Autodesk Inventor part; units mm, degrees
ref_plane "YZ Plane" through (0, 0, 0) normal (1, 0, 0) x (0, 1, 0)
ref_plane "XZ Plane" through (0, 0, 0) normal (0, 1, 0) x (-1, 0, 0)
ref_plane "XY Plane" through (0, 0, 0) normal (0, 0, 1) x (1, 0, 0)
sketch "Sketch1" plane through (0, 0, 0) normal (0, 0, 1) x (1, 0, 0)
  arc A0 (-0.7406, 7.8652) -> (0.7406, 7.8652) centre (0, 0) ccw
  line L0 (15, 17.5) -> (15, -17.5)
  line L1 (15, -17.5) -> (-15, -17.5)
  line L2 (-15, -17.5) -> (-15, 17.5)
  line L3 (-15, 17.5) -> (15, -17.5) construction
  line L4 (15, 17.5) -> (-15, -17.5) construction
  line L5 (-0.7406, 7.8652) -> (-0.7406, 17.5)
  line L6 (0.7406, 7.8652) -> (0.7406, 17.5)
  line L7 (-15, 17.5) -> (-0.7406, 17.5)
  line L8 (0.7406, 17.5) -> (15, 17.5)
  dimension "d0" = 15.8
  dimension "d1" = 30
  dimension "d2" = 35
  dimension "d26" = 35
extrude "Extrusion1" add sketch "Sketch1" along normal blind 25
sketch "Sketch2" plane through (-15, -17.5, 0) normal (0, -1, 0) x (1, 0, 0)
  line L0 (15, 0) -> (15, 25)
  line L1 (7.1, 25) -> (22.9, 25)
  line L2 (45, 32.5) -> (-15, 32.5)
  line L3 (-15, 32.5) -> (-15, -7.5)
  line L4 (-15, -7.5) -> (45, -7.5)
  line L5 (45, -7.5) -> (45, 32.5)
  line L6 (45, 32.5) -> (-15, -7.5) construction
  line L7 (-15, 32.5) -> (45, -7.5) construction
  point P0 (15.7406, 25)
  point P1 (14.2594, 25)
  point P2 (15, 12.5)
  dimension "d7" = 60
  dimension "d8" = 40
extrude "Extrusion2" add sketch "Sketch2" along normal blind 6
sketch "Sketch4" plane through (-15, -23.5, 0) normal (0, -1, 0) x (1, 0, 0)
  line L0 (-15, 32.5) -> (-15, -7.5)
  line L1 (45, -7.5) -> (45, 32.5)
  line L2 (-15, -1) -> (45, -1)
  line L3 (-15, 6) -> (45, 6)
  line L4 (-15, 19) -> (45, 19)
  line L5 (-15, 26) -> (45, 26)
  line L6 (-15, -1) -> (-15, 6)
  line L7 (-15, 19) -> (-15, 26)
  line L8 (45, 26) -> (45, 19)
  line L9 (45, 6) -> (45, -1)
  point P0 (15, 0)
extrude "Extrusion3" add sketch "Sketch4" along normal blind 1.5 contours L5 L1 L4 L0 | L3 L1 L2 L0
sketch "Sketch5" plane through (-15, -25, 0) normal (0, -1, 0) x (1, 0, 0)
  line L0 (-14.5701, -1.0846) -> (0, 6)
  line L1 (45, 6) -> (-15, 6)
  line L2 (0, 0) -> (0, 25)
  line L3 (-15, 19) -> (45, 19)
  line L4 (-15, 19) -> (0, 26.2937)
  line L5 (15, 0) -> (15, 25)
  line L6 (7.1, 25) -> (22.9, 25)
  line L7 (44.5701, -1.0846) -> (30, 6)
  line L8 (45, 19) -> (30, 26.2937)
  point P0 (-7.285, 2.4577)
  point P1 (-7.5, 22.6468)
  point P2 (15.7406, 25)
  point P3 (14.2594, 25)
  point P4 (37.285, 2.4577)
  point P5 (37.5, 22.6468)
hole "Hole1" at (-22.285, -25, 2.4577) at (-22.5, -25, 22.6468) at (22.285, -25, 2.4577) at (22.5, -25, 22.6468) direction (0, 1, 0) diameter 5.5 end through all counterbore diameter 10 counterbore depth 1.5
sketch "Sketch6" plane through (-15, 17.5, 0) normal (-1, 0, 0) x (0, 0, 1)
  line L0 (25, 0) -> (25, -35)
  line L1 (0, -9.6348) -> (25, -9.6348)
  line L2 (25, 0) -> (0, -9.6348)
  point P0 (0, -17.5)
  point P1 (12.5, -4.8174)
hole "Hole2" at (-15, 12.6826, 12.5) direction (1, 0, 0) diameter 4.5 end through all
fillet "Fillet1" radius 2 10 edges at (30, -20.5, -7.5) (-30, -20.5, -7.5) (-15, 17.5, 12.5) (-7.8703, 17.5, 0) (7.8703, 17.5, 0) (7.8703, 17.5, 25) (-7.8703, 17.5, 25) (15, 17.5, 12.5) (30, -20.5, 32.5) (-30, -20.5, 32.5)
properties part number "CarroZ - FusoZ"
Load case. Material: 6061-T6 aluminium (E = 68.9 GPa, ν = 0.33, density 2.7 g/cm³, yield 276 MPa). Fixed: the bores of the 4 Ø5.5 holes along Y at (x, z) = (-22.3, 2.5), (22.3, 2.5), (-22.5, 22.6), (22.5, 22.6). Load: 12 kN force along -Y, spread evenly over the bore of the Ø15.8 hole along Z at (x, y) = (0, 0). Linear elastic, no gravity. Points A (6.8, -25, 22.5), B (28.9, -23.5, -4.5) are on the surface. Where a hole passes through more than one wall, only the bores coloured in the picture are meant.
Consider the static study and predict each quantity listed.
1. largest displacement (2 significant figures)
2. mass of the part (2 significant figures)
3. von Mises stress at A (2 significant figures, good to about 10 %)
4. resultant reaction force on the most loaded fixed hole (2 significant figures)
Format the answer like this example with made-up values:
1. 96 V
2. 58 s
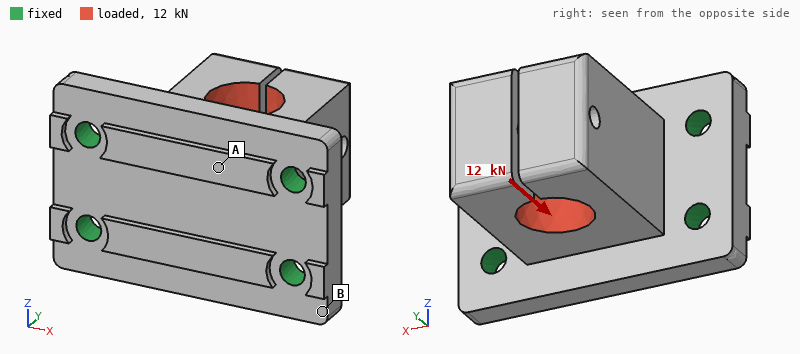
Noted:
1. 0.12 mm
2. 95 g
3. 44 MPa
4. 3.3 kN
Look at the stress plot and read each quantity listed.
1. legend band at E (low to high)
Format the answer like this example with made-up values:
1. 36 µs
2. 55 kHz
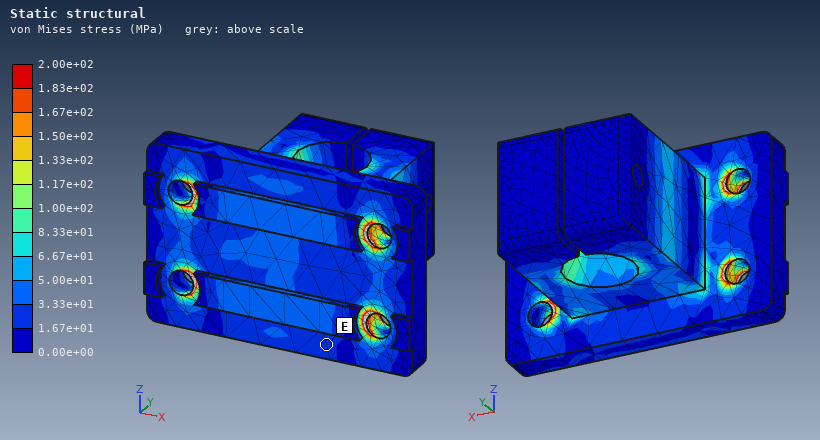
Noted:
1. 1.67e+01 to 3.33e+01 MPa
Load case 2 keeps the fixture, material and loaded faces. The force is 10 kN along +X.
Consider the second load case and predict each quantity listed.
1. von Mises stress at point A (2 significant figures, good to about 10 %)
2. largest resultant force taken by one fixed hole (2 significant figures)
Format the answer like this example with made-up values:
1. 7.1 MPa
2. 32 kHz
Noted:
1. 19 MPa
2. 3.9 kN
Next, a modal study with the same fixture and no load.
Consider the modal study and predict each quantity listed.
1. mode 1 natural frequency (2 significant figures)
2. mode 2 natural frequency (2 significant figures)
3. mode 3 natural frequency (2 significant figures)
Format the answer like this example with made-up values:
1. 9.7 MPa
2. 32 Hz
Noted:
1. 5700 Hz
2. 5800 Hz
3. 6100 Hz
